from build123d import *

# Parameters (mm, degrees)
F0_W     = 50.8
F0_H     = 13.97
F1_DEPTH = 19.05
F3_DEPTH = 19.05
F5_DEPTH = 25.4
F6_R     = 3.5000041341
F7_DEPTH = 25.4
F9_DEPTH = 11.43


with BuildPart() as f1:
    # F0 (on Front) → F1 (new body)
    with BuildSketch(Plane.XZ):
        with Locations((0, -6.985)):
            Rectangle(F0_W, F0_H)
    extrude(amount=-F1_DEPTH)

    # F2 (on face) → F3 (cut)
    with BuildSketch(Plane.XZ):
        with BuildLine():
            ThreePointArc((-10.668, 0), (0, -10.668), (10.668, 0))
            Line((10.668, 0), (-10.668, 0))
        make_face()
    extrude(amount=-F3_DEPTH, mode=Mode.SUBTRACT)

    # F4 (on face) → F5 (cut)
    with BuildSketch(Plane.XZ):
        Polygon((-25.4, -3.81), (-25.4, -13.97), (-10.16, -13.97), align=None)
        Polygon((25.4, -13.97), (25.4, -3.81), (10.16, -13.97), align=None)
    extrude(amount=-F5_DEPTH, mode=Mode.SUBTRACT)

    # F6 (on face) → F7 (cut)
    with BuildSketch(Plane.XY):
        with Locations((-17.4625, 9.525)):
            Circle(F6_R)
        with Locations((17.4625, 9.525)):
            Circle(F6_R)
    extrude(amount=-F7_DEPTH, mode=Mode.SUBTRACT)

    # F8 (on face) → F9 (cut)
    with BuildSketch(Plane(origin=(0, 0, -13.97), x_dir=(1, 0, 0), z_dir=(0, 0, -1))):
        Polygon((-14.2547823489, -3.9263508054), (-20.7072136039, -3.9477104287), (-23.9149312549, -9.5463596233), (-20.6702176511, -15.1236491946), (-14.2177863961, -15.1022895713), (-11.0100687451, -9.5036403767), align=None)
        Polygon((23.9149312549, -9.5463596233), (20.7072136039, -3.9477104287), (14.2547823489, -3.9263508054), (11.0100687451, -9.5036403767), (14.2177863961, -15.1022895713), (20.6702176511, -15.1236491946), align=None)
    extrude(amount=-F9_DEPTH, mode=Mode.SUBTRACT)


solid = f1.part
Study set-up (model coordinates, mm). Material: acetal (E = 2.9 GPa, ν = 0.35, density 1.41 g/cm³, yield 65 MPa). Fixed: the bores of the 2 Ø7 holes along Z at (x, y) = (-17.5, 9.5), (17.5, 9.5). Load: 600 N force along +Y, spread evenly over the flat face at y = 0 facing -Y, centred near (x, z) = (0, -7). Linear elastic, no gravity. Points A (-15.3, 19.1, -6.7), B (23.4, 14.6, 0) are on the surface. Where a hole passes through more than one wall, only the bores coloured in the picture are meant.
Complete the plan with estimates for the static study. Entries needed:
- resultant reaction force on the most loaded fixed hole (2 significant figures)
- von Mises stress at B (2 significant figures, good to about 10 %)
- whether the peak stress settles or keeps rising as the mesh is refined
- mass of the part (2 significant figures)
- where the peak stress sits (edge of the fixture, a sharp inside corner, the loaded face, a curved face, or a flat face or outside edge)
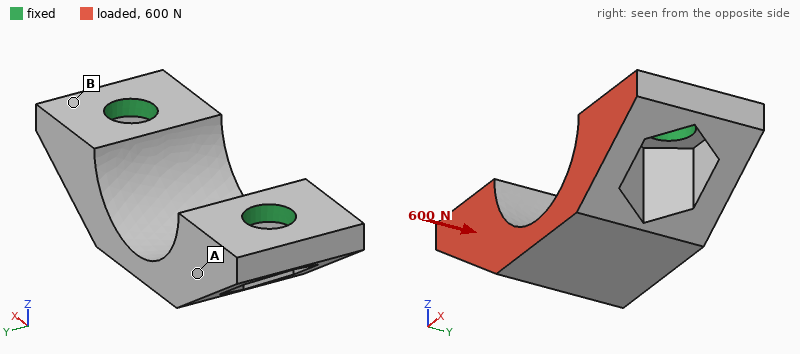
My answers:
300 N
7.6 MPa
keeps rising
7.8 g
edge of the fixture
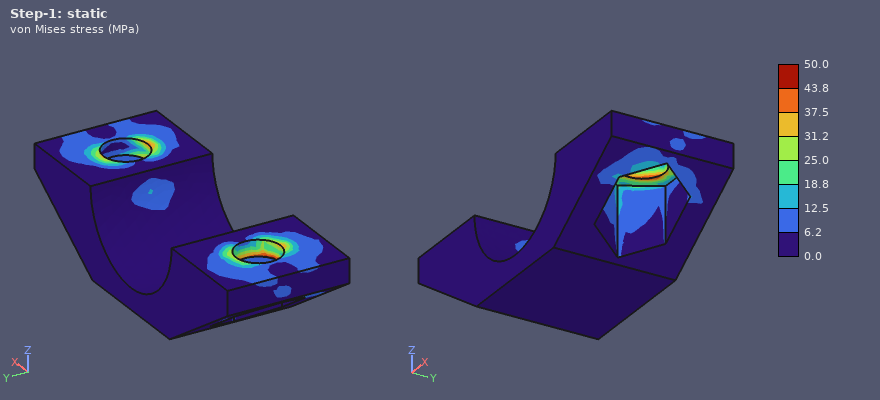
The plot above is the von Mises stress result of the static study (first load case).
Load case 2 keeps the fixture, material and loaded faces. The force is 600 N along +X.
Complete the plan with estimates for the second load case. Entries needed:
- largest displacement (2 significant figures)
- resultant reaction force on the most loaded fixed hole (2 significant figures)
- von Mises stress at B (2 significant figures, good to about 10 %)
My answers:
0.14 mm
320 N
5.6 MPa
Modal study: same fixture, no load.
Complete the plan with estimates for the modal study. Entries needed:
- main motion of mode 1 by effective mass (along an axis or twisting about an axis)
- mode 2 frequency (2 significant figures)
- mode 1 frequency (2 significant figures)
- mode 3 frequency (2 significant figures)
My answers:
along Y
5800 Hz
3000 Hz
5900 Hz
